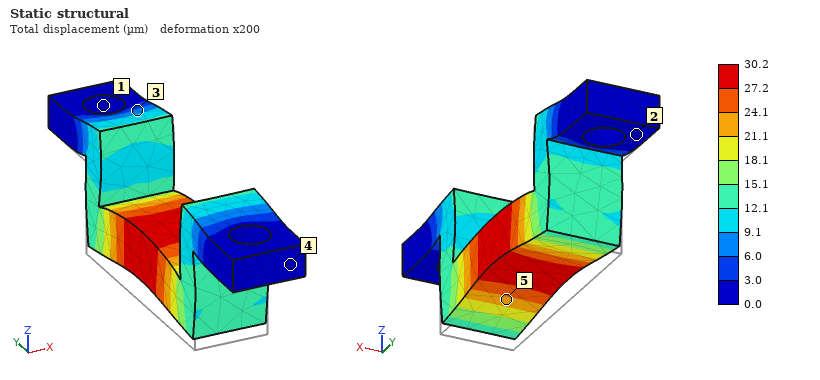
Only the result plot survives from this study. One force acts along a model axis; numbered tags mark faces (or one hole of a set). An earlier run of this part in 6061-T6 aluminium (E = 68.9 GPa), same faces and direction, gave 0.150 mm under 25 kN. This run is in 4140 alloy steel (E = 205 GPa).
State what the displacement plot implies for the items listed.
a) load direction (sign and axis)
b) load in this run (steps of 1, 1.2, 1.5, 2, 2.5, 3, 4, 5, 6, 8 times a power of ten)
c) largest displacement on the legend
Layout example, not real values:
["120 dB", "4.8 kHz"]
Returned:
["+Z", "15 kN", "30.2 µm"]
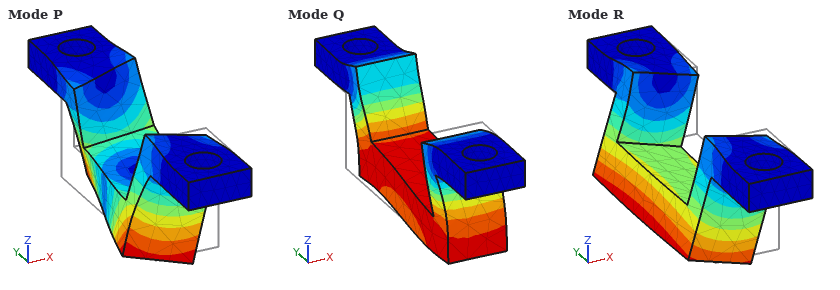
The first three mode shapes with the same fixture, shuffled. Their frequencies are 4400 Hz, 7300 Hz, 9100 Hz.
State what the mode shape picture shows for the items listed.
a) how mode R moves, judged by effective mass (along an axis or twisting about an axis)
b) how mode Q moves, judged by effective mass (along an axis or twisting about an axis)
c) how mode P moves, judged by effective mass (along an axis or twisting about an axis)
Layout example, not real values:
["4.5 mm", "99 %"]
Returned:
["along X", "along Y", "twisting about Z"]
